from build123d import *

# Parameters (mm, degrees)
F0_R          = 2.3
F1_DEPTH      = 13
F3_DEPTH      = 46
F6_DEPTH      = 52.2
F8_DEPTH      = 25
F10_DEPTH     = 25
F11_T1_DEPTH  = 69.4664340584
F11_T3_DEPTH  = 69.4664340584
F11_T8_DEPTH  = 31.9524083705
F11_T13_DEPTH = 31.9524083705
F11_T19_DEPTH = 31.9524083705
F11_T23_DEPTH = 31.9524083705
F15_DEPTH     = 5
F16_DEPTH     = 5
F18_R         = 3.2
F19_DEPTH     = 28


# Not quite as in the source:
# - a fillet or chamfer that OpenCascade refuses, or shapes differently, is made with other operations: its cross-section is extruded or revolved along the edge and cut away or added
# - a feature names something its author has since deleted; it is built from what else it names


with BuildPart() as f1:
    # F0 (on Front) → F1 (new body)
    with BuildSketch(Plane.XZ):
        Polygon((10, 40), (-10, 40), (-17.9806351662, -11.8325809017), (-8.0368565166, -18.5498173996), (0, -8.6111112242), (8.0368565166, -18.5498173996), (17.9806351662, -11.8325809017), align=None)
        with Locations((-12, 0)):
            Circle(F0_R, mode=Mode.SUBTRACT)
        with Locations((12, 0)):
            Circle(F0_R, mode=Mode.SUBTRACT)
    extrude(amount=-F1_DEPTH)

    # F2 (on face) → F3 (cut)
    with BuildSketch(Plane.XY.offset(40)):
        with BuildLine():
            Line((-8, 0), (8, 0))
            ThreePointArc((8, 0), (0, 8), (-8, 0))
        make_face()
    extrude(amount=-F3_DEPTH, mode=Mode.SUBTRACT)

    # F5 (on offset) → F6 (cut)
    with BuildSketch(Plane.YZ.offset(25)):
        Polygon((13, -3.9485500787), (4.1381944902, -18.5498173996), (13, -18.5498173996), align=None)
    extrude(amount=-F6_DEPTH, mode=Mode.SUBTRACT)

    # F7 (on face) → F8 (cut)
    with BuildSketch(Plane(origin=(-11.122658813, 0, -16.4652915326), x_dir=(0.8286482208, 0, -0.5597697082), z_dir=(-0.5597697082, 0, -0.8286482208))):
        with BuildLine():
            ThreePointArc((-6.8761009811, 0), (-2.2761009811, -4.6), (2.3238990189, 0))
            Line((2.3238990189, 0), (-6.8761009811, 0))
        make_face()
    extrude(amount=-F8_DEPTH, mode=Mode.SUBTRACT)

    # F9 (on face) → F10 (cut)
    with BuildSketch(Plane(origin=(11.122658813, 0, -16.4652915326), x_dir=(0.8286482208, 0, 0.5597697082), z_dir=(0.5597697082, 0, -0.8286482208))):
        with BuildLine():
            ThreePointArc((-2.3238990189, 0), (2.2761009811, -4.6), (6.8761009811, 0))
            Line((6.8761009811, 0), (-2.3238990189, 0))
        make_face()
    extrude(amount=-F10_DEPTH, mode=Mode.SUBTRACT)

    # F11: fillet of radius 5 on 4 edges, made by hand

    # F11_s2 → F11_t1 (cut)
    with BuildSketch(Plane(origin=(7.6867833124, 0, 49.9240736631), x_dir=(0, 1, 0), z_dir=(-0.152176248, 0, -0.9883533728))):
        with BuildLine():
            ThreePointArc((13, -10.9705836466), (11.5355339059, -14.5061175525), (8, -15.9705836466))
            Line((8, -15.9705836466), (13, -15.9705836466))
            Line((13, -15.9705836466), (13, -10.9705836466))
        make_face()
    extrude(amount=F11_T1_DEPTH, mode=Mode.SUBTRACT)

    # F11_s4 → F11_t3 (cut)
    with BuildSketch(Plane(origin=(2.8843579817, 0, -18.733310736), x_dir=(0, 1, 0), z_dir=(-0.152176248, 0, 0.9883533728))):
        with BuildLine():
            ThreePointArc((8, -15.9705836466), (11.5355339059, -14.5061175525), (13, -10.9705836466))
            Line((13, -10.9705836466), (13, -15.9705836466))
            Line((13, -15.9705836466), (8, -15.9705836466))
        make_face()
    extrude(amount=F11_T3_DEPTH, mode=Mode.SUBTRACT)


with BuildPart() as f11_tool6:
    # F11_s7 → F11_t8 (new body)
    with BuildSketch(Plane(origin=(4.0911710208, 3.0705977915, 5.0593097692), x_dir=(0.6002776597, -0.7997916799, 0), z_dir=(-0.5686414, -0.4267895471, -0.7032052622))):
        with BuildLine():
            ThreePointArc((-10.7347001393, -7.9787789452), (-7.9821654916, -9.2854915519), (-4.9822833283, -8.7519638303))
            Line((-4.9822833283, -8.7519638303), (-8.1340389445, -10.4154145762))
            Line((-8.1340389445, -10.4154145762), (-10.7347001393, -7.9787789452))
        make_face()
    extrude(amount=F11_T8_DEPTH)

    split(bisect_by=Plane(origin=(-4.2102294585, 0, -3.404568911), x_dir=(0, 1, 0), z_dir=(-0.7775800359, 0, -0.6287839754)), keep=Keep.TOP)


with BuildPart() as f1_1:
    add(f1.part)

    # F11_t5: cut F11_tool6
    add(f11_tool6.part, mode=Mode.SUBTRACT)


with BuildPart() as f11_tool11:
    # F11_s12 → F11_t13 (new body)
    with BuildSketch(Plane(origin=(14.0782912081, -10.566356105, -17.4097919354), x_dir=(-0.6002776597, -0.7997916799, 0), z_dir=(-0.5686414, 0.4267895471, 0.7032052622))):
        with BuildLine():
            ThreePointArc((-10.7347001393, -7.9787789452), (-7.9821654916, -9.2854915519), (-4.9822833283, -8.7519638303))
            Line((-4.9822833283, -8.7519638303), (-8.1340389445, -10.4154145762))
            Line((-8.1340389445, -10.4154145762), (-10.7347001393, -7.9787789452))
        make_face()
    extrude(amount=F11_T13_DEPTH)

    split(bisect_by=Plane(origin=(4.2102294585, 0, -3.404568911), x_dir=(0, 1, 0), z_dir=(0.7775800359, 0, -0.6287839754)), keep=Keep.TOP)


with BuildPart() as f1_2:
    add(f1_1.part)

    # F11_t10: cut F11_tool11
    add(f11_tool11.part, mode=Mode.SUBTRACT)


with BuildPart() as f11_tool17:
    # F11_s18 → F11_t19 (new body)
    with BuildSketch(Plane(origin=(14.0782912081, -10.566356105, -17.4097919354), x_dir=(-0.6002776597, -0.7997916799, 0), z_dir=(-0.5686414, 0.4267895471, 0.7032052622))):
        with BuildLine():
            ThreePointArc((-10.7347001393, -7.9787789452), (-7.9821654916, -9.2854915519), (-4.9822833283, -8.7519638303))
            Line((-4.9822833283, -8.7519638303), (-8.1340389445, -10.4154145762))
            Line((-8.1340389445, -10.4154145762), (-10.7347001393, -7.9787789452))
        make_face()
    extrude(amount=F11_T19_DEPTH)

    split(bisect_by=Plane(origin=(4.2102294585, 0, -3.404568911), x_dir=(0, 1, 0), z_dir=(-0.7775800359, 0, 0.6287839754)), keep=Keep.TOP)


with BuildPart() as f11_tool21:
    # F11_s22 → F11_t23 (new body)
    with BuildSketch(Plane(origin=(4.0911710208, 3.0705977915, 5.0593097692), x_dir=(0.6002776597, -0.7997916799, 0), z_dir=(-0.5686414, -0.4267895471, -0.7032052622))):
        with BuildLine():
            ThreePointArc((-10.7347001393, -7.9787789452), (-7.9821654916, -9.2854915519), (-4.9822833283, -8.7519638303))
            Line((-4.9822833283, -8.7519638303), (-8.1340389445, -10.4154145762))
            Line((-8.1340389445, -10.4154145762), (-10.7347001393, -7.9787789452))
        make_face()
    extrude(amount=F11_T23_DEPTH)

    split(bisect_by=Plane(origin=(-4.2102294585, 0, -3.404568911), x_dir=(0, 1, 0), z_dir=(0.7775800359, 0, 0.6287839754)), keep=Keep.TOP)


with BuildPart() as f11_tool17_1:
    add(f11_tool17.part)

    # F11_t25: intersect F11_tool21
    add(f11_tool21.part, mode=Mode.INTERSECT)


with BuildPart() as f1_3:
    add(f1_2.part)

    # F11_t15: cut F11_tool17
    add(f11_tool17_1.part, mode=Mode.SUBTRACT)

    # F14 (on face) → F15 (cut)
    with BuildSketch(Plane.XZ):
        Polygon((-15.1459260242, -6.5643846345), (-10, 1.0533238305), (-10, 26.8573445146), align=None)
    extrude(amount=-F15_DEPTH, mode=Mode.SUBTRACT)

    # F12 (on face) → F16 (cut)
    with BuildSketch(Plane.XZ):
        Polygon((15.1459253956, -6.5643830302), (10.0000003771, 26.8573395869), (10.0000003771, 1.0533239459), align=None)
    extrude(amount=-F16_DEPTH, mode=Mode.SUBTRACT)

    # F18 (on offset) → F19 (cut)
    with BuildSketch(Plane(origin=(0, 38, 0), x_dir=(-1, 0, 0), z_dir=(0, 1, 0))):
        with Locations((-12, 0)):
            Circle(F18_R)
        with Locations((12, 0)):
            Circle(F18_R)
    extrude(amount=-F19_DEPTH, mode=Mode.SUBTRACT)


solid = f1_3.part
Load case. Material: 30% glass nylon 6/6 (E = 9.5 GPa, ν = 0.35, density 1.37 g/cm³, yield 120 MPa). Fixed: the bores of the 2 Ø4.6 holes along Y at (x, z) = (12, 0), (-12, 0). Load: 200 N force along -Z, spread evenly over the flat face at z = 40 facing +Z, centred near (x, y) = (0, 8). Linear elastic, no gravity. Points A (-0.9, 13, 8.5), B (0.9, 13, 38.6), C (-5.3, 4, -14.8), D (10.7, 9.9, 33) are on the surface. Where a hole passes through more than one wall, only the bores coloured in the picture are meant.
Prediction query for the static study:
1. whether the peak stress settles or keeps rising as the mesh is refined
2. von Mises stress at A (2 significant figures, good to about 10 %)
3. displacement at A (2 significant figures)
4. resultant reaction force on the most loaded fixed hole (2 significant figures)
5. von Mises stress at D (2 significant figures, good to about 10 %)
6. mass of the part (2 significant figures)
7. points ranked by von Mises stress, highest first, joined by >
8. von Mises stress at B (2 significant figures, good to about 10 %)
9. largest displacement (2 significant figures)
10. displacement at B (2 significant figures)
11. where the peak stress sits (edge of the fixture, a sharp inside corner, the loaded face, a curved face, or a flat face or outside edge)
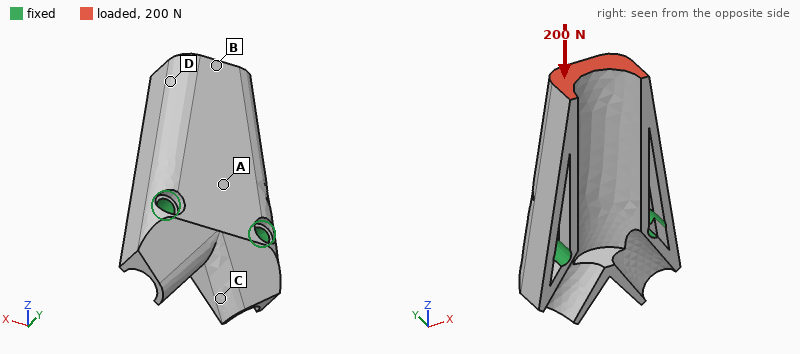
keeps rising
0.66 MPa
2.5 µm
100 N
1.0 MPa
16 g
B > D > A > C
1.4 MPa
9.2 µm
8.8 µm
edge of the fixture
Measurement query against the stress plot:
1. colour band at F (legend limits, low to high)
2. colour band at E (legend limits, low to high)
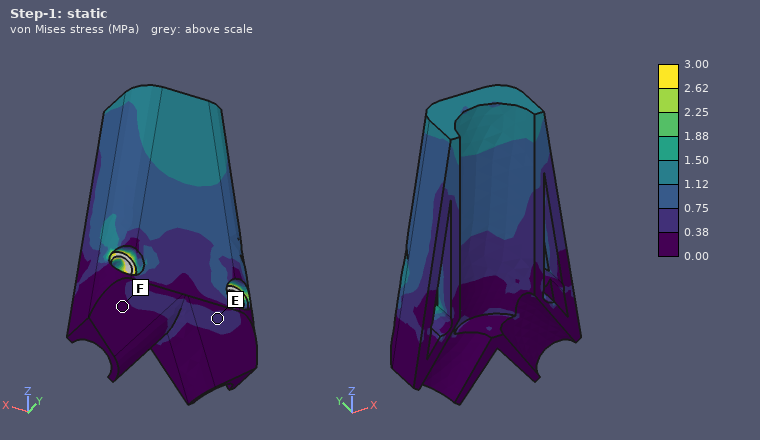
0.00 to 0.38 MPa
0.38 to 0.75 MPa
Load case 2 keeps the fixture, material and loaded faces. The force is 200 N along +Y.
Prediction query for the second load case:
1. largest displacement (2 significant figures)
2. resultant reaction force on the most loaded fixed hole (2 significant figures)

0.25 mm
110 N
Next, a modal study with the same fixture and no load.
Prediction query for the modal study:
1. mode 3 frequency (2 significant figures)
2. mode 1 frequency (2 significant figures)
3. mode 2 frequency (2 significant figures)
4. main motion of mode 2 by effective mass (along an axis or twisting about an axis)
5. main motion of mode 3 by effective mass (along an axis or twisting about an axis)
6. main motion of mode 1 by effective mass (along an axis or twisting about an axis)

8000 Hz
2800 Hz
5100 Hz
along X
along X
along Y
